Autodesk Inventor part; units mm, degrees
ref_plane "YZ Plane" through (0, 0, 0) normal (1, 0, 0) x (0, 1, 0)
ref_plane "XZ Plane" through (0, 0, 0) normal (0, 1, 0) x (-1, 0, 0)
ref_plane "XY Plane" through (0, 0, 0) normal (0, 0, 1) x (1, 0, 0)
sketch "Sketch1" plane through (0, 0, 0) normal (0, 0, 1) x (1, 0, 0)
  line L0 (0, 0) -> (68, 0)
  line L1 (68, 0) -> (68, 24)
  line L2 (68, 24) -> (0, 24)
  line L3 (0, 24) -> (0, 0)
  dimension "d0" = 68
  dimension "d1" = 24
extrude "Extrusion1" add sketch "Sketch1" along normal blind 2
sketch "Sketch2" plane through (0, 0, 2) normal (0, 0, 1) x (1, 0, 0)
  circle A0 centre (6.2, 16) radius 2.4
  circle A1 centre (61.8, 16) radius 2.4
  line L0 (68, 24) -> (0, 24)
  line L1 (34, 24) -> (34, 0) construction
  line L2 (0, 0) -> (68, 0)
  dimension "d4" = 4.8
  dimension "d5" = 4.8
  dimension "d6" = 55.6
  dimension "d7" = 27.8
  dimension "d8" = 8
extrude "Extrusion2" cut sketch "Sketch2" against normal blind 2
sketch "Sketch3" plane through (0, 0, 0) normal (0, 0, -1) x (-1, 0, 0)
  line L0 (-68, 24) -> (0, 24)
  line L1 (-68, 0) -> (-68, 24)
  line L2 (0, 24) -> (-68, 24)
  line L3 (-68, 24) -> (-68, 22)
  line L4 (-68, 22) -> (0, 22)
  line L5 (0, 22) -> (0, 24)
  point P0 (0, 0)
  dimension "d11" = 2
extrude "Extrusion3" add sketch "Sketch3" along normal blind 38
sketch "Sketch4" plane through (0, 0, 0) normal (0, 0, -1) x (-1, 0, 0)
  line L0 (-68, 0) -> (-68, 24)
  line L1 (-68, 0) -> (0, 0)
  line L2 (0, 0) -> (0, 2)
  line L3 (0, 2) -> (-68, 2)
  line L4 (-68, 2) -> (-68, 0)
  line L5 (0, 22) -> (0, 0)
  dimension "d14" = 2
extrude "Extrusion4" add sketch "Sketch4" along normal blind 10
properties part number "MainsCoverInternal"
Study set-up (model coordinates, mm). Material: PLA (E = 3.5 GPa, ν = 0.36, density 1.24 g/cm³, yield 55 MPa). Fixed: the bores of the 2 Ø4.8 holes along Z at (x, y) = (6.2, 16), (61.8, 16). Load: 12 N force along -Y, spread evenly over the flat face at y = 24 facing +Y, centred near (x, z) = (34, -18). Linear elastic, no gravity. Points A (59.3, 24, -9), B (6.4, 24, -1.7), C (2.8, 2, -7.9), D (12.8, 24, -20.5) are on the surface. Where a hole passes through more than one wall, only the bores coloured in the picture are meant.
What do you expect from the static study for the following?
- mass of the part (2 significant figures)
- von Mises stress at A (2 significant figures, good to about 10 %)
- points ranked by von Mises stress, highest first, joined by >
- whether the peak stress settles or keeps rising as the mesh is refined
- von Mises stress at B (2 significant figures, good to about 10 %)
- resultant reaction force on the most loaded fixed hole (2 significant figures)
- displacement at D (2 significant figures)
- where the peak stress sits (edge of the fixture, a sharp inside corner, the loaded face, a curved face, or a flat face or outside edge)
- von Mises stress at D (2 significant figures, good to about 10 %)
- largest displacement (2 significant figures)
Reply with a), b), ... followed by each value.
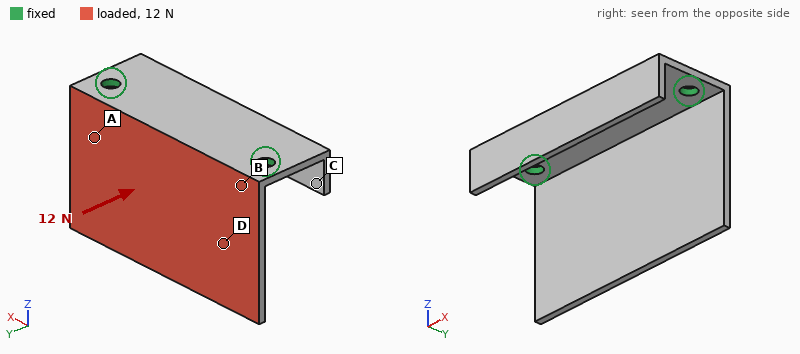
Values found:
a) 12 g
b) 2.7 MPa
c) B > A > D > C
d) keeps rising
e) 4.2 MPa
f) 6.0 N
g) 0.41 mm
h) edge of the fixture
i) 0.97 MPa
j) 0.87 mm
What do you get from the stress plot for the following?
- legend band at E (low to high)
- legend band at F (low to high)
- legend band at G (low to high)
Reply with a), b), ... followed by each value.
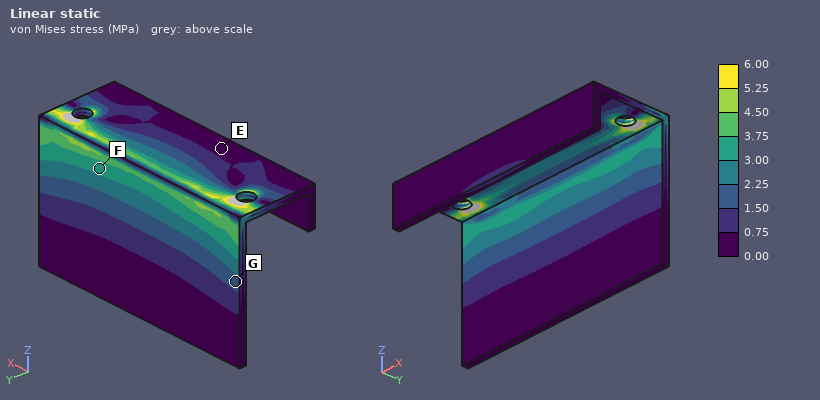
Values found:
a) 0.00 to 0.75 MPa
b) 3.00 to 3.75 MPa
c) 1.50 to 2.25 MPa
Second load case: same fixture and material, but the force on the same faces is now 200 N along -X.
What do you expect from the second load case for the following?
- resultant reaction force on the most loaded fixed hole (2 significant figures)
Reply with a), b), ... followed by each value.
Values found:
a) 120 N
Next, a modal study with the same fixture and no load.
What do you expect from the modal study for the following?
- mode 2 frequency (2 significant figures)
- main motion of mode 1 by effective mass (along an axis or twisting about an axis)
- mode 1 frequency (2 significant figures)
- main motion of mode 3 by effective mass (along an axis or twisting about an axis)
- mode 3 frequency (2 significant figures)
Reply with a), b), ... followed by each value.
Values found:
a) 530 Hz
b) along Y
c) 280 Hz
d) along Z
e) 960 Hz
